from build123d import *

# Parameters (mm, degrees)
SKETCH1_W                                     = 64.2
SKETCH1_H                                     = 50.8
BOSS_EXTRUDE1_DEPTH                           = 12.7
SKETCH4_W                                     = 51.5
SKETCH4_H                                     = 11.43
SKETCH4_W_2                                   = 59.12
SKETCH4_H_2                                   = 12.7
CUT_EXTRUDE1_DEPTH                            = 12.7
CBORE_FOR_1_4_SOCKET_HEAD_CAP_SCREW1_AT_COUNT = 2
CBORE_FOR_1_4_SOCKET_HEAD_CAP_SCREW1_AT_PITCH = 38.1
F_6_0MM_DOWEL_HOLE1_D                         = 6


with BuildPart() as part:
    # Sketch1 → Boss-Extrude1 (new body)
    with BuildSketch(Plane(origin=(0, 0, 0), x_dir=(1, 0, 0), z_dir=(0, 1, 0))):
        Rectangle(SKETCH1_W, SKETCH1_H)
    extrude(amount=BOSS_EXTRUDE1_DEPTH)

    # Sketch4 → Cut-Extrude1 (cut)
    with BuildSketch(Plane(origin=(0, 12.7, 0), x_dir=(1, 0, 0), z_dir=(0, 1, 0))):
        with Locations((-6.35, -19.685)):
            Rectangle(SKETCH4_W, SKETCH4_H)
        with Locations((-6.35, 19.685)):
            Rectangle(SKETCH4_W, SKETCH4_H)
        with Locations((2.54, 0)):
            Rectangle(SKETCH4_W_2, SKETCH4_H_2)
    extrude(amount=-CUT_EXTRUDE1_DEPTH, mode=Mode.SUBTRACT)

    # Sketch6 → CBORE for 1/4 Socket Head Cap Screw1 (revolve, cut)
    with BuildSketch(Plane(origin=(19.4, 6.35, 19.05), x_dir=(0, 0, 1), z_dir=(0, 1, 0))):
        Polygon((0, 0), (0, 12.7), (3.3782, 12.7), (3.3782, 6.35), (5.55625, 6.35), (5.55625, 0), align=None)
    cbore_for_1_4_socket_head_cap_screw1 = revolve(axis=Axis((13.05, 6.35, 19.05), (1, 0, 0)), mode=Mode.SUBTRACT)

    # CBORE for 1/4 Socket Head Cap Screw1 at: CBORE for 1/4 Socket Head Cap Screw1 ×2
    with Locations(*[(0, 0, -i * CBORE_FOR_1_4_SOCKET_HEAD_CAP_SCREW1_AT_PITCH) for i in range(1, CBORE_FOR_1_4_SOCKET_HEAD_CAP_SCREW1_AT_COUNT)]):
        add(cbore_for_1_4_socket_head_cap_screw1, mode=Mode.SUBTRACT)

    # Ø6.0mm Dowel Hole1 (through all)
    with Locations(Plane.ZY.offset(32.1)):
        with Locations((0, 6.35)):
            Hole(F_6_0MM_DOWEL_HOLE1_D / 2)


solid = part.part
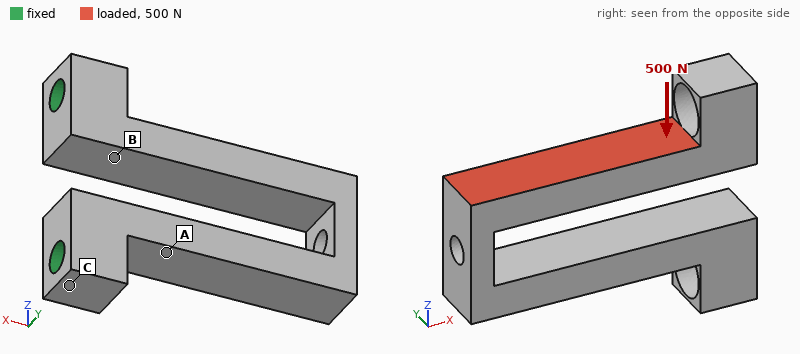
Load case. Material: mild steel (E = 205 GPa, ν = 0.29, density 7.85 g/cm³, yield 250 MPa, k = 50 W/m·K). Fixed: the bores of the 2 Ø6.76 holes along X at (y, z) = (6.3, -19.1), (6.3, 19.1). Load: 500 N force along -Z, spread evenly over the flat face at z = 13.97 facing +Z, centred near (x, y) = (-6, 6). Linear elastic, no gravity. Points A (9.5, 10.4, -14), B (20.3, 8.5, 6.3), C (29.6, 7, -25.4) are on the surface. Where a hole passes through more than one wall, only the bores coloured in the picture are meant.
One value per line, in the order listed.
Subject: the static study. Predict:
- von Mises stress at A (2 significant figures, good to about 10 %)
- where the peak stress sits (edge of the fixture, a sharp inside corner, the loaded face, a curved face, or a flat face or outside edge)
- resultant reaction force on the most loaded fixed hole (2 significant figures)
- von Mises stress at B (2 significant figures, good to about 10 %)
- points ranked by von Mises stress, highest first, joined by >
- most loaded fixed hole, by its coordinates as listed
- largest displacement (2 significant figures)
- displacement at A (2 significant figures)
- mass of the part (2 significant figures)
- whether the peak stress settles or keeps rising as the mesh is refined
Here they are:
18 MPa
a sharp inside corner
460 N
29 MPa
B > A > C
(6.3, 19.1)
33 µm
6.9 µm
120 g
keeps rising
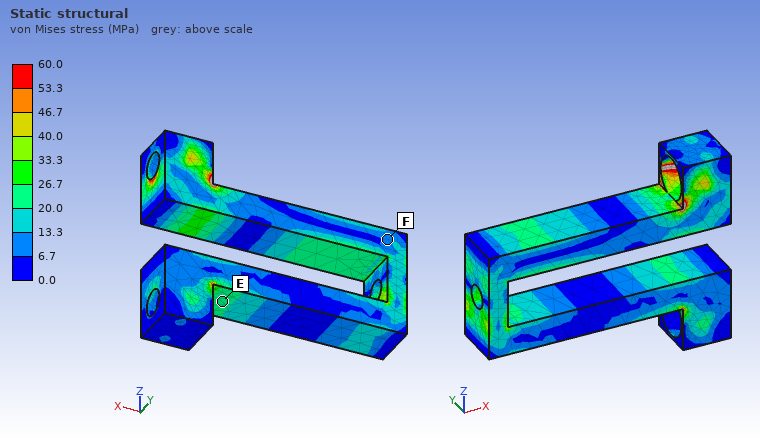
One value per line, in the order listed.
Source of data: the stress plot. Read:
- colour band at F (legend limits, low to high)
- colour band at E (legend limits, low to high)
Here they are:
6.7 to 13.3 MPa
20.0 to 26.7 MPa
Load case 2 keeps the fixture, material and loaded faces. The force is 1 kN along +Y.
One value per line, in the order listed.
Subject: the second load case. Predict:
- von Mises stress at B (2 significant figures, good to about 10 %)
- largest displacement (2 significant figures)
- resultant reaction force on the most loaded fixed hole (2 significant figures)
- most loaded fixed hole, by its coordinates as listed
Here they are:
48 MPa
0.13 mm
800 N
(6.3, 19.1)
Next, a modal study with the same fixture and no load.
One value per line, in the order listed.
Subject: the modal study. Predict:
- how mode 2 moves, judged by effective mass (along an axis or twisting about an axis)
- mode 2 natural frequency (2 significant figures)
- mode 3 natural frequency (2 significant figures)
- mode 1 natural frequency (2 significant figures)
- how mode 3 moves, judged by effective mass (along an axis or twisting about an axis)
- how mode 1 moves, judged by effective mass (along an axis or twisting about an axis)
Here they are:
along Z
2400 Hz
4800 Hz
2000 Hz
twisting about X
along Y
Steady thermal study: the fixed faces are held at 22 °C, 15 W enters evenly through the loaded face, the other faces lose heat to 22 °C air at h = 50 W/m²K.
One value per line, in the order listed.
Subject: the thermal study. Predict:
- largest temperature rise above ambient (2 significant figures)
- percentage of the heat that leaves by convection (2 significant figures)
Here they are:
50 K
38 %
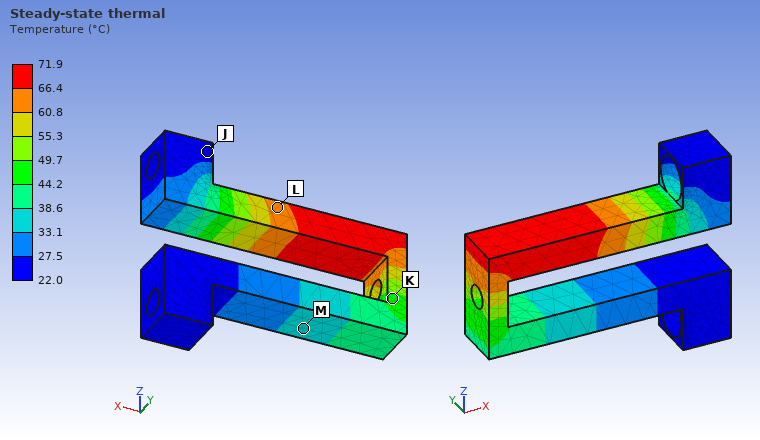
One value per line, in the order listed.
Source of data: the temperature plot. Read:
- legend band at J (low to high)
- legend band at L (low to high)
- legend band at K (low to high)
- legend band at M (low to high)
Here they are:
22.0 to 27.5 °C
60.8 to 66.4 °C
44.2 to 49.7 °C
33.1 to 38.6 °C
